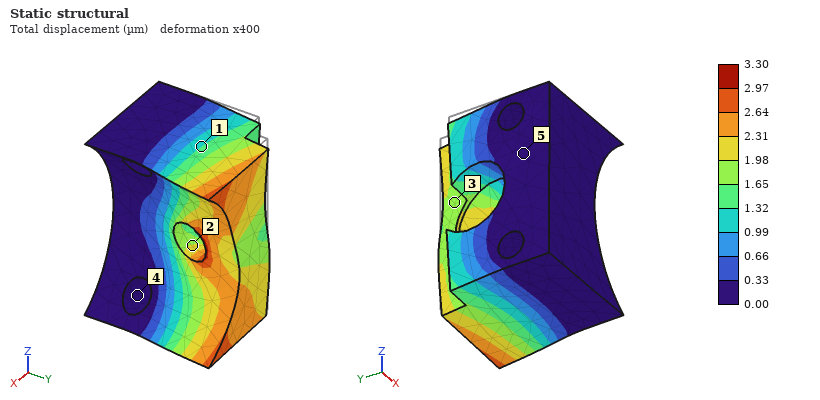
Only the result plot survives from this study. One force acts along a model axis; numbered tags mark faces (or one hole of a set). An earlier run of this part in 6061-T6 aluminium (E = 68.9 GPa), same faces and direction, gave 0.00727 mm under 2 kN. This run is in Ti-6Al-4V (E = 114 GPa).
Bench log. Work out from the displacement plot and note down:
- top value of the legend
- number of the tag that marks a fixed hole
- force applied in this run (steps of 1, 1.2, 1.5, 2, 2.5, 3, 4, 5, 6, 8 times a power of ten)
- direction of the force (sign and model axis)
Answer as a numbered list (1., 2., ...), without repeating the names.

1. 3.30 µm
2. 4
3. 1.5 kN
4. -Z
